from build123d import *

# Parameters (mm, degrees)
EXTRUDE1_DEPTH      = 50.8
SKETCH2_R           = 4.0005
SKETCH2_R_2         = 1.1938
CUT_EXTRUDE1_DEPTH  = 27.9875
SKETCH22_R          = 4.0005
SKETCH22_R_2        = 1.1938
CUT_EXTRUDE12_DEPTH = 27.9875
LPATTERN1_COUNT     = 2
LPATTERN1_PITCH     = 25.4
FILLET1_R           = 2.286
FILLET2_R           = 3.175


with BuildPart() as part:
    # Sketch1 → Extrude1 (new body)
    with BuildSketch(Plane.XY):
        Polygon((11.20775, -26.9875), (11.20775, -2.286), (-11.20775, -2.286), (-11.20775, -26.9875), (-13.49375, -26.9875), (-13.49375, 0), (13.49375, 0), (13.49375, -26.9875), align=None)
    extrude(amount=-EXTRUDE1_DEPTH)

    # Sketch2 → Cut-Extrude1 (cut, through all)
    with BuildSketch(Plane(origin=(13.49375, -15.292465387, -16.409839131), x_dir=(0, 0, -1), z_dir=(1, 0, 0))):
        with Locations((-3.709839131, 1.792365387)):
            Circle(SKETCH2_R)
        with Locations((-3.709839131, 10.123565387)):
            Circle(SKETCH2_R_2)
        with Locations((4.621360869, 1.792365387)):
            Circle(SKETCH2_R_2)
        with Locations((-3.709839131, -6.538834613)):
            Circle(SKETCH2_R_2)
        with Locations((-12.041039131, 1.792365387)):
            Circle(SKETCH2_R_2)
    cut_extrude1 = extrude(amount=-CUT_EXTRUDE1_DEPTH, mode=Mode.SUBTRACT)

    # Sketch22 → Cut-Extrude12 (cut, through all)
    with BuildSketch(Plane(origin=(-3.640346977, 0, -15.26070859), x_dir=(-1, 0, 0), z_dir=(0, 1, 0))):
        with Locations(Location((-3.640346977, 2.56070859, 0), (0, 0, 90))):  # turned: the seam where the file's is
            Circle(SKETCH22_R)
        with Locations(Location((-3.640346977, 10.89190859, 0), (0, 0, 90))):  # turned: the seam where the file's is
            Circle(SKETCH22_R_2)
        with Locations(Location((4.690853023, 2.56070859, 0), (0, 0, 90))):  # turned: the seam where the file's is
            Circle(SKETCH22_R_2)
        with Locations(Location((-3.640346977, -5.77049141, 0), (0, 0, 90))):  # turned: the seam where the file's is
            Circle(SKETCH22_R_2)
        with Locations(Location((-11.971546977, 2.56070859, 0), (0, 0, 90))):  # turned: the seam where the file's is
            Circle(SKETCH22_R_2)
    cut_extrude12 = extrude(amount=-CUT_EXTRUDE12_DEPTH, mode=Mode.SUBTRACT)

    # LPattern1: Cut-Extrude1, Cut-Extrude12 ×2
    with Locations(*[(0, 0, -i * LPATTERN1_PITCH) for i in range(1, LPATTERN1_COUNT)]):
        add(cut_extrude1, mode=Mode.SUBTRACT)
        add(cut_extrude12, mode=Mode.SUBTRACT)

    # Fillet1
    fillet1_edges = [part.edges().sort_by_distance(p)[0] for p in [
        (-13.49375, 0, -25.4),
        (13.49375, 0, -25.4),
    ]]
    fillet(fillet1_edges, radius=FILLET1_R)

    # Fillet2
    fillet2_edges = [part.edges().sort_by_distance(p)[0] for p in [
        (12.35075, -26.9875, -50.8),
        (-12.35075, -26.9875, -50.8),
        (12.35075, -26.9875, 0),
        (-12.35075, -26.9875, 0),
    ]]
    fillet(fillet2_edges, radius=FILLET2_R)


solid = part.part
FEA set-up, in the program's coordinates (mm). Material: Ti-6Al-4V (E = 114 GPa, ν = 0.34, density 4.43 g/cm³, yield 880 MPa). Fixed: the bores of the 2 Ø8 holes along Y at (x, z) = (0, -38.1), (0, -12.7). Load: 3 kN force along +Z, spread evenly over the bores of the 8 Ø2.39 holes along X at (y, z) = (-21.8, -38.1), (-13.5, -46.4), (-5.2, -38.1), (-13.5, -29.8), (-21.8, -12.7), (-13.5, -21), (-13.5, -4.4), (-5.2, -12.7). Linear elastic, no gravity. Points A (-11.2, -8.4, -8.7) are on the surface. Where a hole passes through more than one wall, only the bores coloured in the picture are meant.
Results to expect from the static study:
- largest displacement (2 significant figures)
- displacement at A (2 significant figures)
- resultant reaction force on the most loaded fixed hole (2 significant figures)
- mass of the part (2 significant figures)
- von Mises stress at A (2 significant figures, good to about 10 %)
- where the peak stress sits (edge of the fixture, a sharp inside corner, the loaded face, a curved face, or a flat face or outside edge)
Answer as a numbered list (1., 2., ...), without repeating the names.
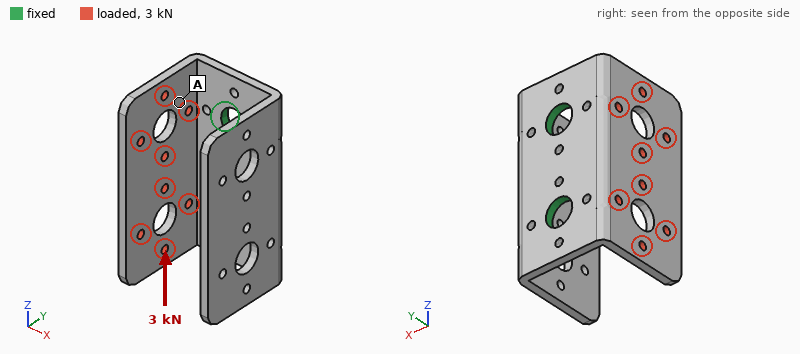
1. 0.37 mm
2. 0.16 mm
3. 2.2 kN
4. 35 g
5. 85 MPa
6. a flat face or outside edge
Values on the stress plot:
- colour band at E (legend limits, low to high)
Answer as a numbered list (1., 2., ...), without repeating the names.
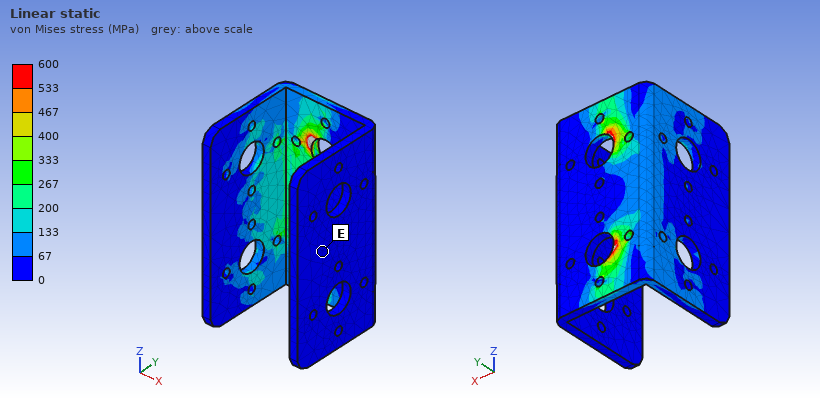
1. 0 to 67 MPa
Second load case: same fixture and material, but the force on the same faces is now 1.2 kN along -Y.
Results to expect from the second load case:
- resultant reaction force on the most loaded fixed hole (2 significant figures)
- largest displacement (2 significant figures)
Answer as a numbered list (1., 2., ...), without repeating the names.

1. 600 N
2. 0.28 mm
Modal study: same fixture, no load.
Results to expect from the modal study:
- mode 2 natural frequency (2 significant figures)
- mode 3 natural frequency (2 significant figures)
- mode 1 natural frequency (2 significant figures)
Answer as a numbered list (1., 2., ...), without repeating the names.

1. 1800 Hz
2. 3100 Hz
3. 1800 Hz
